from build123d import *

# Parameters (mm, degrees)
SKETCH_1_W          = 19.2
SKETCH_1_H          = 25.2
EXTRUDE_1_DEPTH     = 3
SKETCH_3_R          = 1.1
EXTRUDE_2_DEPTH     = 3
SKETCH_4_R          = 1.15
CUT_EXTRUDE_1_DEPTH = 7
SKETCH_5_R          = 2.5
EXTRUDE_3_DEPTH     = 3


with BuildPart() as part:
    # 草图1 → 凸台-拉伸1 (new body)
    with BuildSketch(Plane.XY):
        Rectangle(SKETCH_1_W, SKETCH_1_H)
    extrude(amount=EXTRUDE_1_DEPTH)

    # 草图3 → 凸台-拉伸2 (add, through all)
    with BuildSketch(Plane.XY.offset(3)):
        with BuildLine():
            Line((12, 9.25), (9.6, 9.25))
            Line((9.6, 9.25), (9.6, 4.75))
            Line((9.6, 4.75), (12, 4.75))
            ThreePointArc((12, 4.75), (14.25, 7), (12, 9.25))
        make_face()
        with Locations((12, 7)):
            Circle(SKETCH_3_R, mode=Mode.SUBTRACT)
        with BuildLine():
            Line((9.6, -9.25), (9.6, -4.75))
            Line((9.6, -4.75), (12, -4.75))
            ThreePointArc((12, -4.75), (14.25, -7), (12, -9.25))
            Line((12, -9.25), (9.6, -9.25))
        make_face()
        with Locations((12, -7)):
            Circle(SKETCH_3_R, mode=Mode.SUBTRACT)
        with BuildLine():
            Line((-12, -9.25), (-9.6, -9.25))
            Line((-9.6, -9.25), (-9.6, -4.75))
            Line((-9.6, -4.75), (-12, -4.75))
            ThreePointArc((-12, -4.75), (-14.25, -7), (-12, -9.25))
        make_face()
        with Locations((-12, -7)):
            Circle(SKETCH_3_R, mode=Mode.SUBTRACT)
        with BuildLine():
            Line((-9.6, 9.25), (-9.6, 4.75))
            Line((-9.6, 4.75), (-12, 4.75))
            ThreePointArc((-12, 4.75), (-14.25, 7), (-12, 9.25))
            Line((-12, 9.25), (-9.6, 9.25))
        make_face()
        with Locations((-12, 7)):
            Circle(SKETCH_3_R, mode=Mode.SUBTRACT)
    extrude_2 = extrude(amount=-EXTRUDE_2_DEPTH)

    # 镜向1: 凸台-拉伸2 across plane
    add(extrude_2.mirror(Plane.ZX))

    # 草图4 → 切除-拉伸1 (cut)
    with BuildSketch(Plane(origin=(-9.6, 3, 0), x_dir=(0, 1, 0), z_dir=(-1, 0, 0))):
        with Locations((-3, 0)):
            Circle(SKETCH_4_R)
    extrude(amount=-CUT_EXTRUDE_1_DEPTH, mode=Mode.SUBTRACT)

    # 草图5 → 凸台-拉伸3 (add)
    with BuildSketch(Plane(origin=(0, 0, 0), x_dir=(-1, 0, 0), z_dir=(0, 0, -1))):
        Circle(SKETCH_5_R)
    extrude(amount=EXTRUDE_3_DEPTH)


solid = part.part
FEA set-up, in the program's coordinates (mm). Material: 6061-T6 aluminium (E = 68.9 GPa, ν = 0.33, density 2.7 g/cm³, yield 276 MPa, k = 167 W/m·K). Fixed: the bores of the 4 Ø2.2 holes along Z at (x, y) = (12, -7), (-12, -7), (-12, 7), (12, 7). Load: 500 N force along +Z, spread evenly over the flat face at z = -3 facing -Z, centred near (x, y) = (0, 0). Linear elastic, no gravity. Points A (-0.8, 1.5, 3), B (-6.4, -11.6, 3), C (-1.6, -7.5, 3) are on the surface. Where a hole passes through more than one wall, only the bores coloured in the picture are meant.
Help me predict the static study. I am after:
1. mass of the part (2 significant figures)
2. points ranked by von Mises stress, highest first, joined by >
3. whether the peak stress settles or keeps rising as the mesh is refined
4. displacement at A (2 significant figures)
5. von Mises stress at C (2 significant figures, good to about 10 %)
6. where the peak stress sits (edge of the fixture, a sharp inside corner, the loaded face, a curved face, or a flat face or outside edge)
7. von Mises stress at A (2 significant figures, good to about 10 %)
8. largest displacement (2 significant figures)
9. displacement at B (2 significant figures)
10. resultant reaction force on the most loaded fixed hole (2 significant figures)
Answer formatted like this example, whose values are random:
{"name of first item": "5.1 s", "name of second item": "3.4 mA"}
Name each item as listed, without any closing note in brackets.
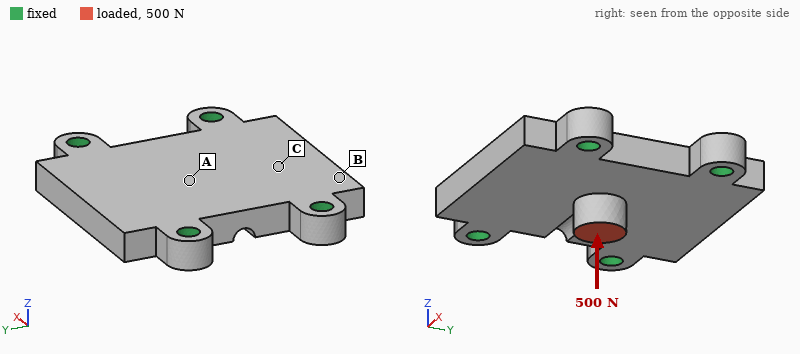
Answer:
{"mass of the part": "4.5 g", "points ranked by von Mises stress, highest first, joined by >": "A > C > B", "whether the peak stress settles or keeps rising as the mesh is refined": "keeps rising", "displacement at A": "18 µm", "von Mises stress at C": "28 MPa", "where the peak stress sits": "a sharp inside corner", "von Mises stress at A": "53 MPa", "largest displacement": "20 µm", "displacement at B": "3.4 µm", "resultant reaction force on the most loaded fixed hole": "130 N"}
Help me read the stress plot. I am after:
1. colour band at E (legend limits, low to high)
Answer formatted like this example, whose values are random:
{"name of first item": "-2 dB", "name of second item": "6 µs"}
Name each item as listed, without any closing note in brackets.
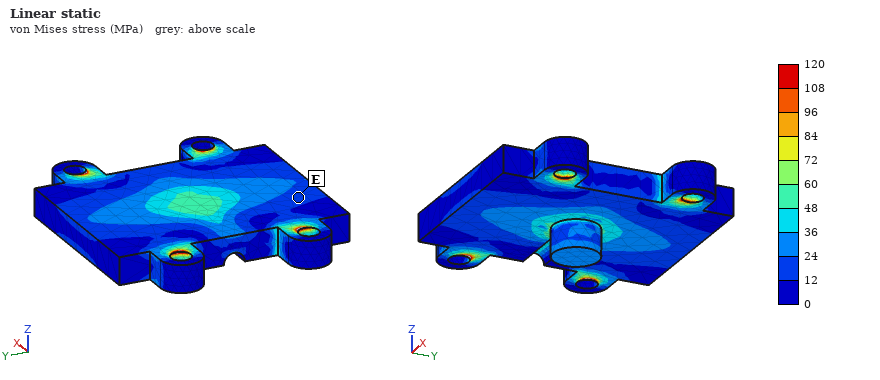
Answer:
{"colour band at E": "12 to 24 MPa"}
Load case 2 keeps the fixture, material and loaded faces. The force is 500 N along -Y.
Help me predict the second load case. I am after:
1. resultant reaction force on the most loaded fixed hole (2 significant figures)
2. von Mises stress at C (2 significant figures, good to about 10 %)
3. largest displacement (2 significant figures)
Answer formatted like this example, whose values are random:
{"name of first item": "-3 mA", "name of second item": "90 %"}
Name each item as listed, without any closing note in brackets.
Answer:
{"resultant reaction force on the most loaded fixed hole": "160 N", "von Mises stress at C": "20 MPa", "largest displacement": "21 µm"}
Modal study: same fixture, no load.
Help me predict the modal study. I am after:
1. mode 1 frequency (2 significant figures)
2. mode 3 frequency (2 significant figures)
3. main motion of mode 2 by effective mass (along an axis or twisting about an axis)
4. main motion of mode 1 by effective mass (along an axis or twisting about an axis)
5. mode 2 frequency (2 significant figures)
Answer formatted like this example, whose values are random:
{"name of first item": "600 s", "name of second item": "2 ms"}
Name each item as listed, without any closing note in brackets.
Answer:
{"mode 1 frequency": "20 kHz", "mode 3 frequency": "31 kHz", "main motion of mode 2 by effective mass": "twisting about X", "main motion of mode 1 by effective mass": "along Z", "mode 2 frequency": "23 kHz"}
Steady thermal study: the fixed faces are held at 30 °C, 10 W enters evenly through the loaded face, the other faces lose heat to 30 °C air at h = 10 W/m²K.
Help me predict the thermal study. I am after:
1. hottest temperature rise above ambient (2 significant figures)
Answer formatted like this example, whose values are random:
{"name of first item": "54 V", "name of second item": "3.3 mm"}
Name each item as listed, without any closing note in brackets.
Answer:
{"hottest temperature rise above ambient": "21 K"}
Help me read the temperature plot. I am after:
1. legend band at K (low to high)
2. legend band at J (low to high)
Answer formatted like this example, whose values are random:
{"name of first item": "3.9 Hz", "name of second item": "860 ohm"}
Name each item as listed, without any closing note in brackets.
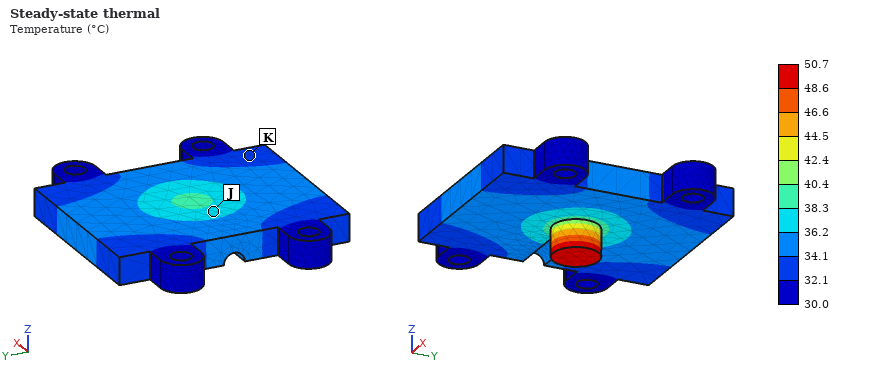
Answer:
{"legend band at K": "32.1 to 34.1 °C", "legend band at J": "36.2 to 38.3 °C"}
